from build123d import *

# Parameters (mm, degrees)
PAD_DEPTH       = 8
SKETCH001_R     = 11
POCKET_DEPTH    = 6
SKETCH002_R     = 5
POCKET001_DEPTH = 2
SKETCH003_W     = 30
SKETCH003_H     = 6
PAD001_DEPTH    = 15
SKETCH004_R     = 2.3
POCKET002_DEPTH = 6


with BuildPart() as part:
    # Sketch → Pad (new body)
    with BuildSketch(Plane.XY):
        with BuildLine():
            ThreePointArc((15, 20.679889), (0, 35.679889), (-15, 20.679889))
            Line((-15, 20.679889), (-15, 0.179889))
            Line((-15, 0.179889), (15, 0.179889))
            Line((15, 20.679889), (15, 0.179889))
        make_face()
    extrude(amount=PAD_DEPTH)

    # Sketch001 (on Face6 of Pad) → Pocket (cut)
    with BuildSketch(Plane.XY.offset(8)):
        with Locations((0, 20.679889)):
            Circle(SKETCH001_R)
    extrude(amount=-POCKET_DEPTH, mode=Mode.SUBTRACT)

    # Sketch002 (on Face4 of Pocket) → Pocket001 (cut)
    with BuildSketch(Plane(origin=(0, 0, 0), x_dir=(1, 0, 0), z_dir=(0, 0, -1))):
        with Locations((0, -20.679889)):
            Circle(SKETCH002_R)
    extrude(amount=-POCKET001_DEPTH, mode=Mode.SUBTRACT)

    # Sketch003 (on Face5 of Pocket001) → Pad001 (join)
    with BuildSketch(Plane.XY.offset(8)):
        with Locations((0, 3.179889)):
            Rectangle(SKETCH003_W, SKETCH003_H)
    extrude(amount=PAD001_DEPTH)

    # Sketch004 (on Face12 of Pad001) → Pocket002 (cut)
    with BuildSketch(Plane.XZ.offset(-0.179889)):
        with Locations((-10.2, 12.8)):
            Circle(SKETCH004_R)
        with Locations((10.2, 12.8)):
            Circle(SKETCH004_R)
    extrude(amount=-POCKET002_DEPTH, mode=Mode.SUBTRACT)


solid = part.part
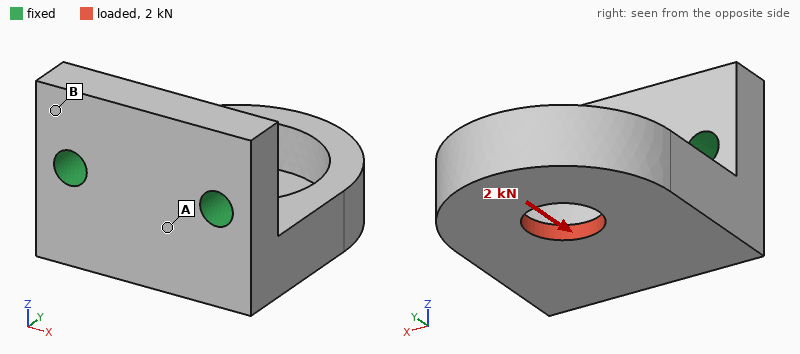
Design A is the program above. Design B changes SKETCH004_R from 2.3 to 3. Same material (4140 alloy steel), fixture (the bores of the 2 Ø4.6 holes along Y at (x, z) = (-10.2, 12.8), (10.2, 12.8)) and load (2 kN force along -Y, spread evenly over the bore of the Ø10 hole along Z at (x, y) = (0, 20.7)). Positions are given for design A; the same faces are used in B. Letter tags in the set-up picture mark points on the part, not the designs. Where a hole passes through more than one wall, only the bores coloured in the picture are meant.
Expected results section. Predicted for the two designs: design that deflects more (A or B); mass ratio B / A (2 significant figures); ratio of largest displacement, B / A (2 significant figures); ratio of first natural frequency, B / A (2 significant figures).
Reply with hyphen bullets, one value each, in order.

- A
- 0.98
- 0.85
- 1.0
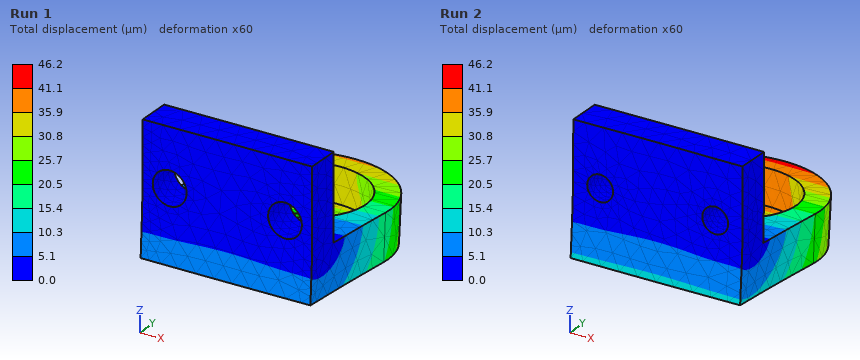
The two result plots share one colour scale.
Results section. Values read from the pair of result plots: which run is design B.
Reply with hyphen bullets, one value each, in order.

- Run 1
